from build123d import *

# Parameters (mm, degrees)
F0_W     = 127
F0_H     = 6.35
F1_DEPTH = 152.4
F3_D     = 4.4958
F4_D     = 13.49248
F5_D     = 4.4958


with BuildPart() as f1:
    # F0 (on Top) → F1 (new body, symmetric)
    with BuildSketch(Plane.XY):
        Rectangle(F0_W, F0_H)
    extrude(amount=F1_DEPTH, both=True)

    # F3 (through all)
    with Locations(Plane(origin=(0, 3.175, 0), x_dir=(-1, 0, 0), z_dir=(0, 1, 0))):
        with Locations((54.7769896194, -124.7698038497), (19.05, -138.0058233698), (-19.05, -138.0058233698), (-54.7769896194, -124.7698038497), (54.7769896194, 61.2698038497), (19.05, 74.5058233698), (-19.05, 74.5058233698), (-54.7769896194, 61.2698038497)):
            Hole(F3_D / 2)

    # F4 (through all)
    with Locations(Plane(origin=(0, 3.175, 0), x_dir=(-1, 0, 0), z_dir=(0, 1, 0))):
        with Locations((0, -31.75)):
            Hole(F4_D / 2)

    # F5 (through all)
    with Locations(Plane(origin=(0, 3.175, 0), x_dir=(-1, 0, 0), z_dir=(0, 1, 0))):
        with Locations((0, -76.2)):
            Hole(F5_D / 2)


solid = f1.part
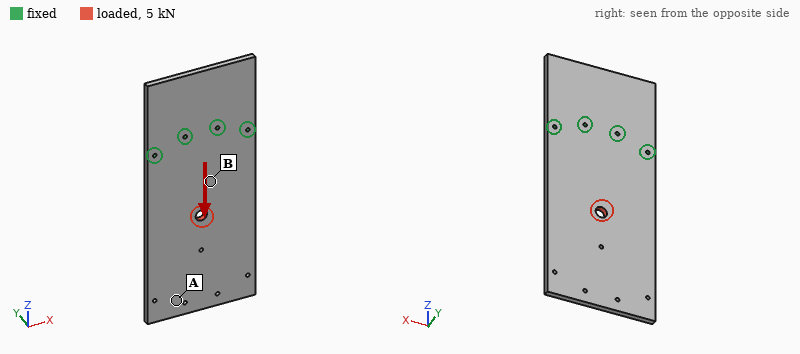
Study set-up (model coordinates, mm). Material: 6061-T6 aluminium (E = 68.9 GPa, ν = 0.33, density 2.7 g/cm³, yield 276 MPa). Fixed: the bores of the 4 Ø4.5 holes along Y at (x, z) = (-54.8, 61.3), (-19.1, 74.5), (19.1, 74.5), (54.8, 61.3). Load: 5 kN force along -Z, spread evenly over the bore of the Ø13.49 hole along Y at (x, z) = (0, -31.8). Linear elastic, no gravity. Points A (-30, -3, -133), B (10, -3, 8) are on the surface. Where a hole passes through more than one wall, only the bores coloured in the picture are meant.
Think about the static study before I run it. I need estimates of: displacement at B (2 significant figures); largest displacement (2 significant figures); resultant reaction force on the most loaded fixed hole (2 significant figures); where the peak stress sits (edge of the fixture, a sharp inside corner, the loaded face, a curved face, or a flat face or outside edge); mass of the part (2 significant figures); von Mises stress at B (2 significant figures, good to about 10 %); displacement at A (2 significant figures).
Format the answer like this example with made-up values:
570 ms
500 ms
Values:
7.0 µm
15 µm
1.3 kN
the loaded face
660 g
8.6 MPa
9.7 µm
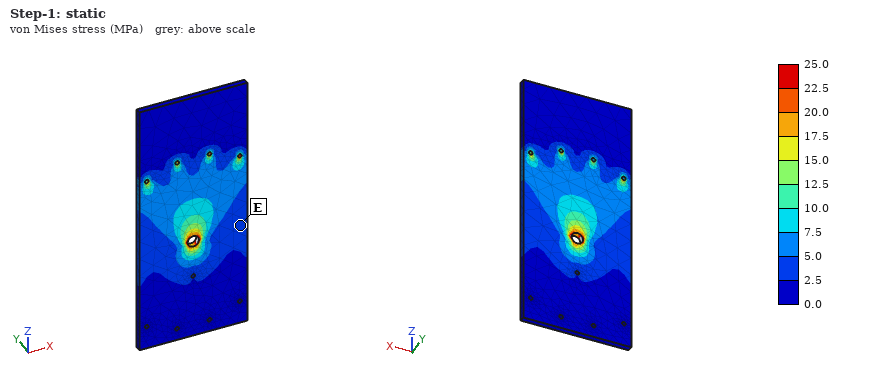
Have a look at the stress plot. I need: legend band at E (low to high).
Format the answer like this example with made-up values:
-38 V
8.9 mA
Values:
2.5 to 5.0 MPa
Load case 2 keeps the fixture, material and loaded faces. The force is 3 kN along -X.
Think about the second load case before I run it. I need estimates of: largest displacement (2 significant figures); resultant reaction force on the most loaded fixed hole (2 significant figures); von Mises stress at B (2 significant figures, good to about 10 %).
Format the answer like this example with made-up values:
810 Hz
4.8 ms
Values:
54 µm
2.6 kN
8.8 MPa
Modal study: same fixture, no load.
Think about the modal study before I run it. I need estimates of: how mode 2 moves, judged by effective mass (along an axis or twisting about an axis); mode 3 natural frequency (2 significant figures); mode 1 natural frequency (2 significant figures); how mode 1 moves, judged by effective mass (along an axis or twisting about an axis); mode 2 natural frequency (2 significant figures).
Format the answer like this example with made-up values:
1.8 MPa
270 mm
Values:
twisting about Z
670 Hz
110 Hz
along Y
420 Hz
